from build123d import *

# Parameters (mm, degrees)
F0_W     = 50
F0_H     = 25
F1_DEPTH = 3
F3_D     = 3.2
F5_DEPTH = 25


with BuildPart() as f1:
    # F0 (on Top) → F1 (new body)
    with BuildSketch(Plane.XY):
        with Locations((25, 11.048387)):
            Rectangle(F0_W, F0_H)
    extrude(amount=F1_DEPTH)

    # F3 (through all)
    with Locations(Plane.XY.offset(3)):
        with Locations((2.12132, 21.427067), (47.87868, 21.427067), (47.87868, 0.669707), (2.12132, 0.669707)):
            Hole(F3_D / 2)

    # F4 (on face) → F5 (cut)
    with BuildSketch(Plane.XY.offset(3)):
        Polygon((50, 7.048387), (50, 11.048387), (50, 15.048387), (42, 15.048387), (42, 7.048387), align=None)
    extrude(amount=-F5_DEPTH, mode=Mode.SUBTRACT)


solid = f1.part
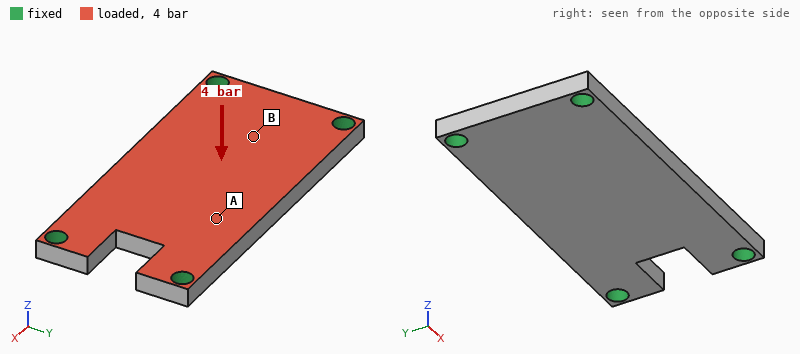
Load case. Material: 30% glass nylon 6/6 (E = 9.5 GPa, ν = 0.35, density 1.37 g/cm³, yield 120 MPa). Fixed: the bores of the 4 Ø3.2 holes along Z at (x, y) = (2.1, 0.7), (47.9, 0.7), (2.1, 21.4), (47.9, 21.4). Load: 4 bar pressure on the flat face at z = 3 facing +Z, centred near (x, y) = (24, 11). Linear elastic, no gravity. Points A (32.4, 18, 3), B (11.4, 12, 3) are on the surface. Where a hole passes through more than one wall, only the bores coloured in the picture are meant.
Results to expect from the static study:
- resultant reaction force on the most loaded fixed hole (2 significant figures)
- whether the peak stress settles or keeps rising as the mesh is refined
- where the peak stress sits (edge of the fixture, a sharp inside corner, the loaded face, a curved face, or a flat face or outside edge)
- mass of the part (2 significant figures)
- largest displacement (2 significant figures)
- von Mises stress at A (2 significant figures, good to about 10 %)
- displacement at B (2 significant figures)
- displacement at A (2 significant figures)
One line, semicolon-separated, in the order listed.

120 N; keeps rising; edge of the fixture; 4.7 g; 0.26 mm; 17 MPa; 0.12 mm; 0.20 mm
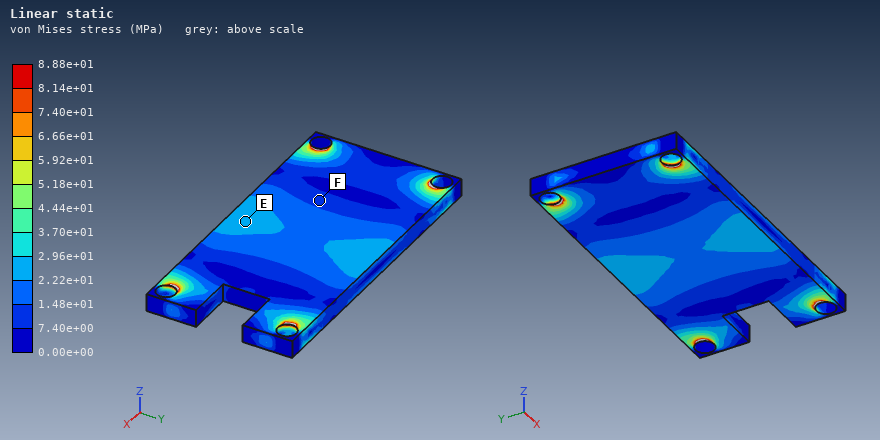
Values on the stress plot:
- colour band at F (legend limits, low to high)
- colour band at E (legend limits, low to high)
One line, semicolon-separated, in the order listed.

7.40e+00 to 1.48e+01 MPa; 2.22e+01 to 2.96e+01 MPa
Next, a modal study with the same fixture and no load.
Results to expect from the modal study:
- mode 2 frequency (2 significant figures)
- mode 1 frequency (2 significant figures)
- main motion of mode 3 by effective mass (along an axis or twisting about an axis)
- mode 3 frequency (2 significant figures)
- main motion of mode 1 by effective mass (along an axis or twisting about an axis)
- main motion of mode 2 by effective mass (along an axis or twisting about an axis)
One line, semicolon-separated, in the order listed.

5900 Hz; 3600 Hz; twisting about Y; 9700 Hz; along Z; twisting about X
